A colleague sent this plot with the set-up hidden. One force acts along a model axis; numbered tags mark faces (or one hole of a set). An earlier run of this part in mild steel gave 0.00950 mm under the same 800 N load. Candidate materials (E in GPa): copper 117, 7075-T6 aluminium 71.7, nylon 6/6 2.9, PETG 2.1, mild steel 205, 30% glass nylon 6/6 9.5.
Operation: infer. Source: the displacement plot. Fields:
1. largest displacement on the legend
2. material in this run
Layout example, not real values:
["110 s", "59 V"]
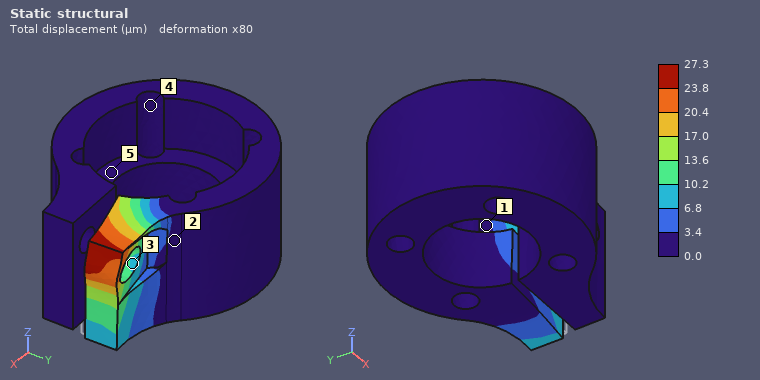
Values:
["27.3 µm", "7075-T6 aluminium"]
